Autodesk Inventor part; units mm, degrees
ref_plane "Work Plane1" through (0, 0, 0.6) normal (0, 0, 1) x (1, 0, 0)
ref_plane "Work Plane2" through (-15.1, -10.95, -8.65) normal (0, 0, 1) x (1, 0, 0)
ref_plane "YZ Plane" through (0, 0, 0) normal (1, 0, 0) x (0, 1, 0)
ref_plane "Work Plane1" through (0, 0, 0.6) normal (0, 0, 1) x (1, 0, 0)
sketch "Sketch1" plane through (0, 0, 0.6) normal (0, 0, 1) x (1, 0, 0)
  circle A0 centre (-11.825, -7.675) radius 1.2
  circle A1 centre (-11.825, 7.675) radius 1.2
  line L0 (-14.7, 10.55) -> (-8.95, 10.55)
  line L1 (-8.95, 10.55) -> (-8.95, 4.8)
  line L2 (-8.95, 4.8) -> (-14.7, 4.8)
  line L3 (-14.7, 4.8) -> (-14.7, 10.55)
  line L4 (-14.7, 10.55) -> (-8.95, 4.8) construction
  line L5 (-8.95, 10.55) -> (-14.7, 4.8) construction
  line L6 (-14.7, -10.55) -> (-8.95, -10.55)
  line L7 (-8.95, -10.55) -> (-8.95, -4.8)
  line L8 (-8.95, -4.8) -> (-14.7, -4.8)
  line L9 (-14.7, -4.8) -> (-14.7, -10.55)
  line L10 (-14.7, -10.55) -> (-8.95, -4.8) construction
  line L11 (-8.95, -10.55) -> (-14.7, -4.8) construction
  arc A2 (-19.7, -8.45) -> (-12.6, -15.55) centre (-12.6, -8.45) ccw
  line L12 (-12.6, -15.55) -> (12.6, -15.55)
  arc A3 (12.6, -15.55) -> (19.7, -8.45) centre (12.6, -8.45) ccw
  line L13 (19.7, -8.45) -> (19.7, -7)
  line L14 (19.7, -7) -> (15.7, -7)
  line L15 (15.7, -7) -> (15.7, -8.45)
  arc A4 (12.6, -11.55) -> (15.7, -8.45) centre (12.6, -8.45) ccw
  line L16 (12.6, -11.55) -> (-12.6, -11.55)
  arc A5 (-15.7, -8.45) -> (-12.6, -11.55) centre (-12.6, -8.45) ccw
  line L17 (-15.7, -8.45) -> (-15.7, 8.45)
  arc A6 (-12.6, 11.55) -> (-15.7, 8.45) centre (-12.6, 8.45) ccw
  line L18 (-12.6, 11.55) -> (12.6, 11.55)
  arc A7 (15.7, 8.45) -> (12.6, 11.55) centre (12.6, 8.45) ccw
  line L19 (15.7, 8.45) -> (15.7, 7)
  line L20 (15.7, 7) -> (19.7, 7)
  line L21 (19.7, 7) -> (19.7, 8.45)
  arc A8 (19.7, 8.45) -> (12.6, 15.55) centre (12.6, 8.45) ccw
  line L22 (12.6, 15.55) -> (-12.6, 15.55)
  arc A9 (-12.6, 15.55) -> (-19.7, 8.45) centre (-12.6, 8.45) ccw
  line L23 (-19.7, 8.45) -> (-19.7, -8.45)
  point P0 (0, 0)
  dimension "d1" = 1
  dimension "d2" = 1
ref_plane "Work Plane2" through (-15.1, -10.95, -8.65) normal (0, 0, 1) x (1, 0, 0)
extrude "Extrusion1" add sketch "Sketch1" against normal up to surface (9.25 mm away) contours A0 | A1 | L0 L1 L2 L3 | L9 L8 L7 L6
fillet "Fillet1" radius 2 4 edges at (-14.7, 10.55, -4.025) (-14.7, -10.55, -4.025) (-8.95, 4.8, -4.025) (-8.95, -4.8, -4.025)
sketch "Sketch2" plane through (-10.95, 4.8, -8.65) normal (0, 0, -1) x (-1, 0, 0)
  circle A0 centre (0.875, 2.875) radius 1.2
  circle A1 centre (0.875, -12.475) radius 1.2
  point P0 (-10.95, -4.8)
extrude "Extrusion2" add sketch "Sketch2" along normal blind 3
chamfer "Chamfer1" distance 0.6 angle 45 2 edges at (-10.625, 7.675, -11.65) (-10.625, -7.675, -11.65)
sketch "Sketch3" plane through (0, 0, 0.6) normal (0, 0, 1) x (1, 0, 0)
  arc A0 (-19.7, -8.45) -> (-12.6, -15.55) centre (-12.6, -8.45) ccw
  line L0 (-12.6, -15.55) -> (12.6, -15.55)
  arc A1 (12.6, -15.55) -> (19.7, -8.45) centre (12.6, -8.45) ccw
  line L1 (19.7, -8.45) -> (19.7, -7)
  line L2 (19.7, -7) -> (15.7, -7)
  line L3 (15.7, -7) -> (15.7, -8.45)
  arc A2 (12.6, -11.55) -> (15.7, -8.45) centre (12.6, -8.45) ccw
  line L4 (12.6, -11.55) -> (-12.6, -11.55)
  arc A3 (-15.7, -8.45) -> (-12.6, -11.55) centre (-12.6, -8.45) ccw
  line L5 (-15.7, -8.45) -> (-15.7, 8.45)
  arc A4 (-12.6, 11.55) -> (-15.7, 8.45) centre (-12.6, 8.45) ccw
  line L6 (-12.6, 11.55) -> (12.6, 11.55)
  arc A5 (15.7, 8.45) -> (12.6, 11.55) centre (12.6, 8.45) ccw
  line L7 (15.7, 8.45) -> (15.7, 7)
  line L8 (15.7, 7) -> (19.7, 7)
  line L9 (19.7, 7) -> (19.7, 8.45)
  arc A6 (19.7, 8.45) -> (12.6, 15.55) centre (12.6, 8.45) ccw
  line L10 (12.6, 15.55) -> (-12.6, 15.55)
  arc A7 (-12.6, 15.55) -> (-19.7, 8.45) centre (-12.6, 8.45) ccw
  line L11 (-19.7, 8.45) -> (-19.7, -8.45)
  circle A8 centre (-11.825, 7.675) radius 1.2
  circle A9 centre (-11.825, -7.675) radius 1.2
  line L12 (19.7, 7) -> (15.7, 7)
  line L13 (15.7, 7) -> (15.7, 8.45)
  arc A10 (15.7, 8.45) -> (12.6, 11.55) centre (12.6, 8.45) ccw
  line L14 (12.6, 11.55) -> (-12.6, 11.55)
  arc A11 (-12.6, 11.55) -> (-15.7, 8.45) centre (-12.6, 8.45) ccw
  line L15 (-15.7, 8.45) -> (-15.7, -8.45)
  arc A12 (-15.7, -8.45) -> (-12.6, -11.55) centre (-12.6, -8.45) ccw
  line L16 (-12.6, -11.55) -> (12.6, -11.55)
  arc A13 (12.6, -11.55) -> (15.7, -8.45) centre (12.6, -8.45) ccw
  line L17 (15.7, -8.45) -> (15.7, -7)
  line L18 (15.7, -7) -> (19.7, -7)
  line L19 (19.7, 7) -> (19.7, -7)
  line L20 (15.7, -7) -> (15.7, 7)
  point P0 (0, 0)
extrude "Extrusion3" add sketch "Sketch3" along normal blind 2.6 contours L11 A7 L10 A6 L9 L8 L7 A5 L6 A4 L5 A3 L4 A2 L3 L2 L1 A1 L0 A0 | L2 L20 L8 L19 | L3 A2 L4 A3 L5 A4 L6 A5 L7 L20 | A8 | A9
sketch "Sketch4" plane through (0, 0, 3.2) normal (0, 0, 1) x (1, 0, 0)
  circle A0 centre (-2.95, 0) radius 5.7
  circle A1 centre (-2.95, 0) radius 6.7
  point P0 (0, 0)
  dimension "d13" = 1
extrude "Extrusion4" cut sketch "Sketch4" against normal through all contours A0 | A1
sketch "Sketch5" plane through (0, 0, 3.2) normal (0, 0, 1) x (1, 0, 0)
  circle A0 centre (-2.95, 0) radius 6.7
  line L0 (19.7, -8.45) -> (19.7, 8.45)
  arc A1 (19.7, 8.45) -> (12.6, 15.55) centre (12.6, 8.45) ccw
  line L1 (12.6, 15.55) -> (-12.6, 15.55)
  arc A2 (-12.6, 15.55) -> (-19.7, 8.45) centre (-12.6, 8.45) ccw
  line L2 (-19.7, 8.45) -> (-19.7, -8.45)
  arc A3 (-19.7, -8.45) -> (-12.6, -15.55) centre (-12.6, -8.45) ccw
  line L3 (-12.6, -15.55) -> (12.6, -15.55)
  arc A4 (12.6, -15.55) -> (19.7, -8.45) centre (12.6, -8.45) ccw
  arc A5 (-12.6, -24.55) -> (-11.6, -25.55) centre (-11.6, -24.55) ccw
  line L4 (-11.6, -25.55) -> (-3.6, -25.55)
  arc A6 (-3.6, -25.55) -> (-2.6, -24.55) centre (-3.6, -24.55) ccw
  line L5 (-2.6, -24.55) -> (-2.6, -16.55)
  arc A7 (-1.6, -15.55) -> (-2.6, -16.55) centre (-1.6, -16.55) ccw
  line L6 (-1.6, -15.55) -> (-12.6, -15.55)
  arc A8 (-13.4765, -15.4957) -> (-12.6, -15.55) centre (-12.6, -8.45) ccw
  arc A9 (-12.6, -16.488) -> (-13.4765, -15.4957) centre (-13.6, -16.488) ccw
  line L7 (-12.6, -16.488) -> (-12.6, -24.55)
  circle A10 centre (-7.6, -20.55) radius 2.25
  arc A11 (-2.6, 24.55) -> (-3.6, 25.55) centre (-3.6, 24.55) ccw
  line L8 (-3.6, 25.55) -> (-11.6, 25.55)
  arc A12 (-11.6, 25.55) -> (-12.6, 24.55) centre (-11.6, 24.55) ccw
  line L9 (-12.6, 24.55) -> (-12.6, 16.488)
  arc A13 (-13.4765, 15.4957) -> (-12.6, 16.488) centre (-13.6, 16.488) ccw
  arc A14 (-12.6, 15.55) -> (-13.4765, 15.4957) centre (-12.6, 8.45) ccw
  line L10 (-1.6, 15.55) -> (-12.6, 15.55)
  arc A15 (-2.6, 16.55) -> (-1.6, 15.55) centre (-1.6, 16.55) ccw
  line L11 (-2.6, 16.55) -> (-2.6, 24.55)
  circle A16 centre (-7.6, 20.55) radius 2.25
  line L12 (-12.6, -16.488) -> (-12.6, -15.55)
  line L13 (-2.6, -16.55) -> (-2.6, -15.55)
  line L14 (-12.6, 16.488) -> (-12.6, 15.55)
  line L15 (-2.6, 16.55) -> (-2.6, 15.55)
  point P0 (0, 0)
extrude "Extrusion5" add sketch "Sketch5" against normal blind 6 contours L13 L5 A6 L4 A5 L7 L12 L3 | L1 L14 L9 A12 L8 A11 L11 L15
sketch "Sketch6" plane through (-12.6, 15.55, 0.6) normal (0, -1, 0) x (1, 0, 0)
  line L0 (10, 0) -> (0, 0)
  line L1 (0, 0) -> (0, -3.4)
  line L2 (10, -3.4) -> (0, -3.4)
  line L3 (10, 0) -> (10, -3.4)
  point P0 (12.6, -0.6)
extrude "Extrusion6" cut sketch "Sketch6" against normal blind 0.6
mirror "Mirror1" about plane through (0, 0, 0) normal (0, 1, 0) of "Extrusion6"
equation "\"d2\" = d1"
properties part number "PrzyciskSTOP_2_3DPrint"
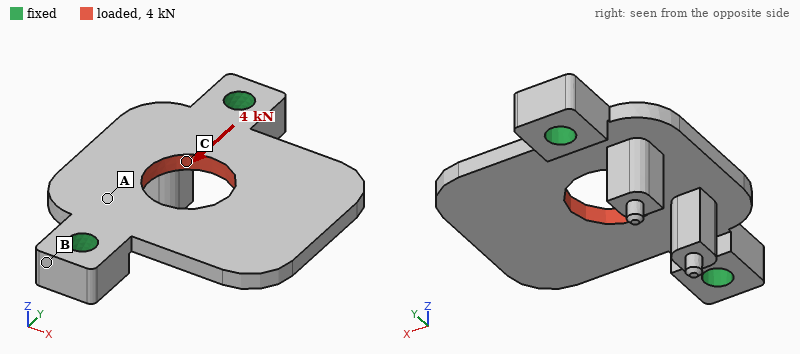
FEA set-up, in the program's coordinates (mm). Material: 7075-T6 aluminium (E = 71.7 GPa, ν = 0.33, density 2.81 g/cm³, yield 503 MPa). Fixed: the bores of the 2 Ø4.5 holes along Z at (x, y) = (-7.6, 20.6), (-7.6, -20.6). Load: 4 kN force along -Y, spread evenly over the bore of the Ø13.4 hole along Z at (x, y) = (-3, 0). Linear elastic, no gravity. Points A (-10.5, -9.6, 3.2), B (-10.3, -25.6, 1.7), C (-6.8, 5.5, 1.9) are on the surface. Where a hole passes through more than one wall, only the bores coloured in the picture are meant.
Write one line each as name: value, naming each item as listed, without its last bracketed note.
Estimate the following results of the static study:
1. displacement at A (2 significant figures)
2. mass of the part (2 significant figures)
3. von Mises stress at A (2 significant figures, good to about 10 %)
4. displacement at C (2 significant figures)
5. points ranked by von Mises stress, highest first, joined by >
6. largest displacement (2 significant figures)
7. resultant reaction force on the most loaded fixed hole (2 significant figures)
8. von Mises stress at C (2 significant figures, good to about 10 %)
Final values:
displacement at A: 6.5 µm
mass of the part: 12 g
von Mises stress at A: 37 MPa
displacement at C: 11 µm
points ranked by von Mises stress, highest first, joined by >: C > A > B
largest displacement: 29 µm
resultant reaction force on the most loaded fixed hole: 2.1 kN
von Mises stress at C: 68 MPa
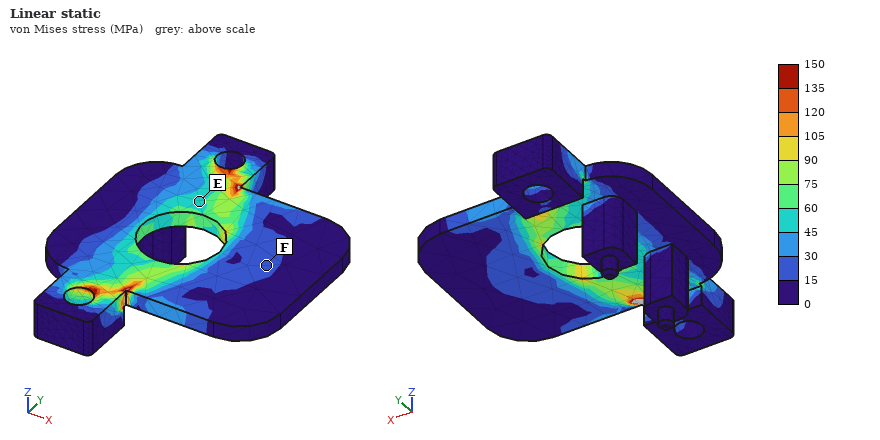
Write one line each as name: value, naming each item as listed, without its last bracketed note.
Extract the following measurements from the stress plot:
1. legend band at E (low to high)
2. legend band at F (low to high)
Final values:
legend band at E: 45 to 60 MPa
legend band at F: 15 to 30 MPa
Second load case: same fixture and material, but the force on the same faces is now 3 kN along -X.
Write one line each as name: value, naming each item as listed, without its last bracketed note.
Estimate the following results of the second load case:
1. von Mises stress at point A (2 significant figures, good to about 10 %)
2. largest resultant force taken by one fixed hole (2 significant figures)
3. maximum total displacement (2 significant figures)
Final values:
von Mises stress at point A: 35 MPa
largest resultant force taken by one fixed hole: 1.5 kN
maximum total displacement: 29 µm
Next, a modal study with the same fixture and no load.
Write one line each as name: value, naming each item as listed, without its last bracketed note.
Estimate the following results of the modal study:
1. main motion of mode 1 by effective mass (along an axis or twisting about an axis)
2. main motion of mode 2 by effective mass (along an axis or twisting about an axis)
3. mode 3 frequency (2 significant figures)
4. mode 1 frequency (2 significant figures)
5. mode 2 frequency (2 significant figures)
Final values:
main motion of mode 1 by effective mass: along Z
main motion of mode 2 by effective mass: along Z
mode 3 frequency: 6800 Hz
mode 1 frequency: 2300 Hz
mode 2 frequency: 6400 Hz
